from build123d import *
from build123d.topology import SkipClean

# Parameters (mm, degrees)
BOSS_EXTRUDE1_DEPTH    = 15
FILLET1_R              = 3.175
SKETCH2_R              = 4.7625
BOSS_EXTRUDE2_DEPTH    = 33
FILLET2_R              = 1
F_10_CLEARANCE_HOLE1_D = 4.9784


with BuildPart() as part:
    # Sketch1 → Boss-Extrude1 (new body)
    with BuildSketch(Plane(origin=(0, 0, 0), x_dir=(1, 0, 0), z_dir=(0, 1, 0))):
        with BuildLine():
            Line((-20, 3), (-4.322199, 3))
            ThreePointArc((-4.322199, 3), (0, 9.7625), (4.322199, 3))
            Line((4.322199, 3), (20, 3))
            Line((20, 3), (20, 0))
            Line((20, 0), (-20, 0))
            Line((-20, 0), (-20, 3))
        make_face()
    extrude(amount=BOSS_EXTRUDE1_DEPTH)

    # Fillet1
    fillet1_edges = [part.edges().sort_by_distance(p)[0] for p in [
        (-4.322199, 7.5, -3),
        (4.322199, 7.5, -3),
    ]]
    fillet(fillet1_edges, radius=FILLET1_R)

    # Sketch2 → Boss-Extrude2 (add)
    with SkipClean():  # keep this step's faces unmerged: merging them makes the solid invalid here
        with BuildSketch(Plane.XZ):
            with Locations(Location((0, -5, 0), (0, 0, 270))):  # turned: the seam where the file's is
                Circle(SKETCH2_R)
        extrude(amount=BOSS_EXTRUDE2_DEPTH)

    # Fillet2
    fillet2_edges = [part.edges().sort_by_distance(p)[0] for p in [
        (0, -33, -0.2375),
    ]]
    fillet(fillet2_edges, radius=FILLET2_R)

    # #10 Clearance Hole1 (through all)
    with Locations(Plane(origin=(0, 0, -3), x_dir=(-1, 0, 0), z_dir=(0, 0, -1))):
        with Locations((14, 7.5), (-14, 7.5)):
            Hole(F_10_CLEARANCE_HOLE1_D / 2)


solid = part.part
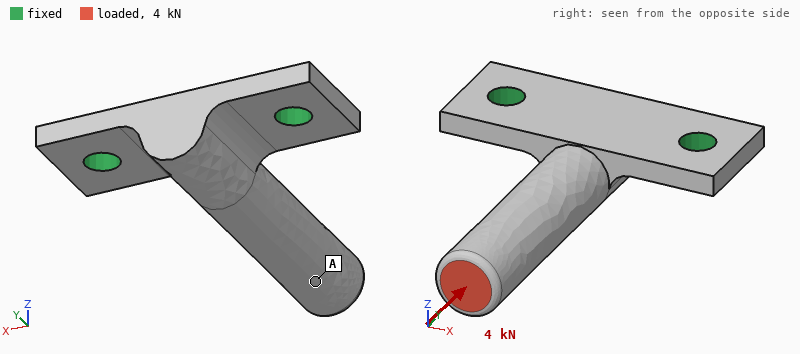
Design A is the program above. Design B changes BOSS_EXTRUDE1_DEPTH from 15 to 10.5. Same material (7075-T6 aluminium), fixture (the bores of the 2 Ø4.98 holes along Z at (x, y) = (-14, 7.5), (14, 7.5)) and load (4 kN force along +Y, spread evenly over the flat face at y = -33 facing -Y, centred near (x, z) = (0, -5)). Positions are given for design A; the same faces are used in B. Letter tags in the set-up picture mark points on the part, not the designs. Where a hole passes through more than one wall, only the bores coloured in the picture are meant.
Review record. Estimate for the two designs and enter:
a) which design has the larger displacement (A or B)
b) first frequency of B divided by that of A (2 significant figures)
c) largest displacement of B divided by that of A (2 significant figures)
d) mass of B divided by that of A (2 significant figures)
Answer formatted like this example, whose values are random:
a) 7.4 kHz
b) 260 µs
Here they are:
a) B
b) 0.84
c) 1.6
d) 0.84
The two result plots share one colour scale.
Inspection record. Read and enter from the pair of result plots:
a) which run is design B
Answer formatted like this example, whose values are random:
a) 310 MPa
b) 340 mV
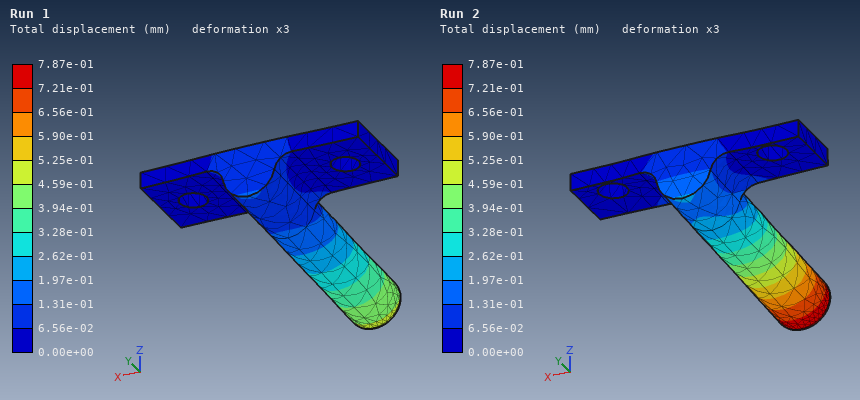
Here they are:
a) Run 2
